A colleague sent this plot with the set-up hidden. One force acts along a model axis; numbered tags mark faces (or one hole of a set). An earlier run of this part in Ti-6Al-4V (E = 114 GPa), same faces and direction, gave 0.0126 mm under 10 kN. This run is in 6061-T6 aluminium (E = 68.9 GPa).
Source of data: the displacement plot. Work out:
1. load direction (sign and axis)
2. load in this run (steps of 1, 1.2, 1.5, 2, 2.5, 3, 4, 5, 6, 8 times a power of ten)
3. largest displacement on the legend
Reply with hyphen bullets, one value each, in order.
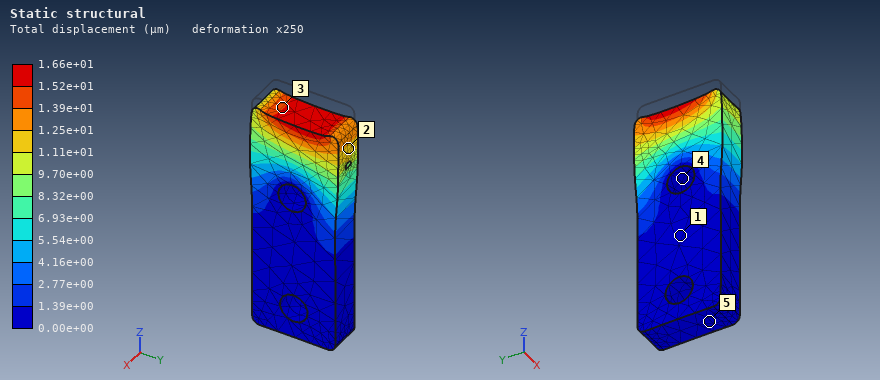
- -Z
- 8 kN
- 1.66e+01 µm
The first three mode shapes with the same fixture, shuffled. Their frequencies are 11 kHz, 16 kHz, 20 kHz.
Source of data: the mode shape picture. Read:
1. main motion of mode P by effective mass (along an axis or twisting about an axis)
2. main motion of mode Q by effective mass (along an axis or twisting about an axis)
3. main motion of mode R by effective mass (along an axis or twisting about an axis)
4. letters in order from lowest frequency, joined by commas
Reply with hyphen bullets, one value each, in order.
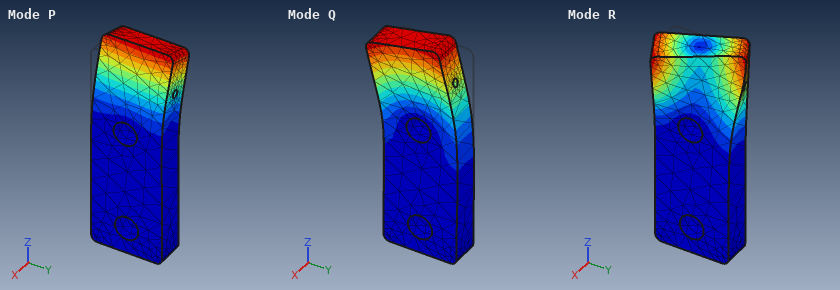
- along X
- along Y
- twisting about Z
- P, Q, R
